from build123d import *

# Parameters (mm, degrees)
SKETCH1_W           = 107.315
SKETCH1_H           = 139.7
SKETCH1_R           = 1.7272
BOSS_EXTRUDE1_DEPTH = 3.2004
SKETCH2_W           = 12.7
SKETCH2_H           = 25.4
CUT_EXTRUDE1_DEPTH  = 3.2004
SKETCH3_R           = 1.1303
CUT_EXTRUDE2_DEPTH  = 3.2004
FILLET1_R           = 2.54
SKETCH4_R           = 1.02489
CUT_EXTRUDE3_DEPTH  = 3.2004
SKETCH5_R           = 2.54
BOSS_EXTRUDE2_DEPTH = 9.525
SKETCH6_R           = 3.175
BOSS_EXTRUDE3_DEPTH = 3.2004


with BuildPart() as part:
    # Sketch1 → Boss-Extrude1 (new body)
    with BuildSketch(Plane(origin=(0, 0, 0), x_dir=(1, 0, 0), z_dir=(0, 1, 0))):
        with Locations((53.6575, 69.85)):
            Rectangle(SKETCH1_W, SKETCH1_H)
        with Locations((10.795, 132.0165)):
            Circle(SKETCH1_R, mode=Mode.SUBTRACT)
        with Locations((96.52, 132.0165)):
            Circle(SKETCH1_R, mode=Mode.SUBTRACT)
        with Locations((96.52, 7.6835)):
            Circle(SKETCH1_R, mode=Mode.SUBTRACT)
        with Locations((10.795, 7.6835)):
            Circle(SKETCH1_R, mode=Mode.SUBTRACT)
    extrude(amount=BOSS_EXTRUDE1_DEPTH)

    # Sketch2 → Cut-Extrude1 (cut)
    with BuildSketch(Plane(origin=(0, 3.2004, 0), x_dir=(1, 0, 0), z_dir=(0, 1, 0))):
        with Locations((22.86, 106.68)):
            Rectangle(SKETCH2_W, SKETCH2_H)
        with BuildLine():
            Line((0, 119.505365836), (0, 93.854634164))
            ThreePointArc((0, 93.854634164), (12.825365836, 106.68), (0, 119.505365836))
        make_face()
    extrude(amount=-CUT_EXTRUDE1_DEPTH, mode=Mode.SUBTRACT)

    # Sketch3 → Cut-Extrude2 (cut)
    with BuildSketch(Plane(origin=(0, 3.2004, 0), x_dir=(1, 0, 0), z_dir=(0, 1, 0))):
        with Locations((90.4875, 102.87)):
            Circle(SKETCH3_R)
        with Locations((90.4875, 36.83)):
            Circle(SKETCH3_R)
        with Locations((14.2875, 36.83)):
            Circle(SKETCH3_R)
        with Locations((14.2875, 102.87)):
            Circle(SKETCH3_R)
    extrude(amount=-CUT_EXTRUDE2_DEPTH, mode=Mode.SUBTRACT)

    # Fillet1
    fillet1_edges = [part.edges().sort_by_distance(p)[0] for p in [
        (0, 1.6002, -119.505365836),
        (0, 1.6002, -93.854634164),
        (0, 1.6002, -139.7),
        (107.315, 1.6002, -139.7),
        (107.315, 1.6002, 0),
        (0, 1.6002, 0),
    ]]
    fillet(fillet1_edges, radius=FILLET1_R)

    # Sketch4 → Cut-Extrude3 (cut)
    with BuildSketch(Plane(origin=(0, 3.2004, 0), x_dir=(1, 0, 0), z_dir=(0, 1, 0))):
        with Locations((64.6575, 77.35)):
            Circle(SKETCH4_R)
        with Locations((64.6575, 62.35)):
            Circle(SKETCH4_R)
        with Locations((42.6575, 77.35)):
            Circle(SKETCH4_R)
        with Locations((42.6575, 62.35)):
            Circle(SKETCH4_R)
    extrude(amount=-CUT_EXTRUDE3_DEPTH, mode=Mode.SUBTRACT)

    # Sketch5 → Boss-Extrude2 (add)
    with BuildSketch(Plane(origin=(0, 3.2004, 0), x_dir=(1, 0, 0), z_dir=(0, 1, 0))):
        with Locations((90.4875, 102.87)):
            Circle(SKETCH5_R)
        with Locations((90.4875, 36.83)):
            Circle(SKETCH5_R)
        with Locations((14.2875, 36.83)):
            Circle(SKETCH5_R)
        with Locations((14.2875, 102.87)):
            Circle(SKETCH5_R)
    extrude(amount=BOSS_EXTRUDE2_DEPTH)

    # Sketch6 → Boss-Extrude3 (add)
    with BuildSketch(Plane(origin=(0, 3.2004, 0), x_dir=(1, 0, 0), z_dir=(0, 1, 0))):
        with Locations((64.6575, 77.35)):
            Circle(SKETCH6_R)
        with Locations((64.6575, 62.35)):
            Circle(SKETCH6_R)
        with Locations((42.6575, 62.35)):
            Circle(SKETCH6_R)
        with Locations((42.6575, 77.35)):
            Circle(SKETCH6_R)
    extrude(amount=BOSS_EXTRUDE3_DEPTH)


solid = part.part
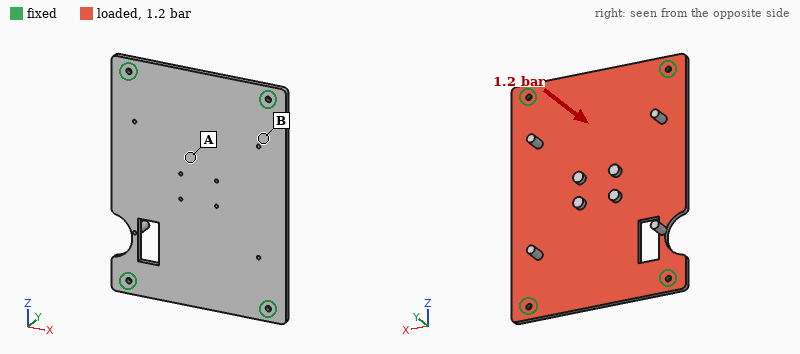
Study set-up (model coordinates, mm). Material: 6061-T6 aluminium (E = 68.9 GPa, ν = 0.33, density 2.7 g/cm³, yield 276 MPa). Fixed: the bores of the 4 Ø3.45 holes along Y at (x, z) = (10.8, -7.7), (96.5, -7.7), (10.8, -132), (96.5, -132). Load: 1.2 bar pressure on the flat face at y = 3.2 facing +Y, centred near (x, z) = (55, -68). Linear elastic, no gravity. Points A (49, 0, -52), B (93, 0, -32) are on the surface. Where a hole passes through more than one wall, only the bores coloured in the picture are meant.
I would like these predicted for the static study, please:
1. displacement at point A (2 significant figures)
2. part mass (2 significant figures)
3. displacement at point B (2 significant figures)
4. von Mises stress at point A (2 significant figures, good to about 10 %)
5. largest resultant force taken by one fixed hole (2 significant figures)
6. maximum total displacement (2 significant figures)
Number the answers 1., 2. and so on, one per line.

1. 0.58 mm
2. 130 g
3. 0.26 mm
4. 41 MPa
5. 440 N
6. 0.65 mm
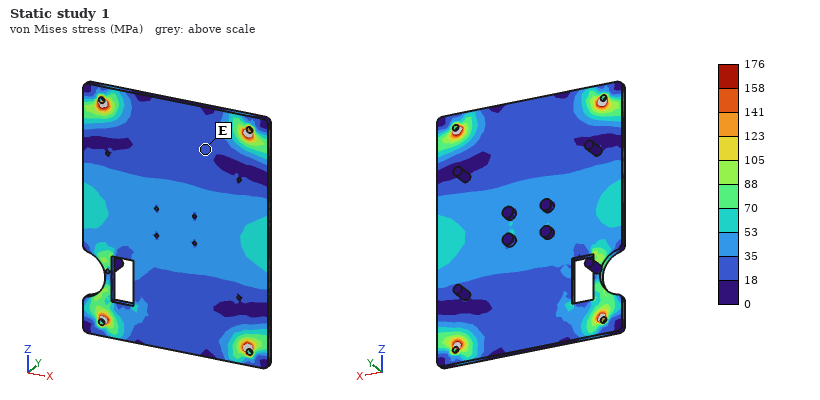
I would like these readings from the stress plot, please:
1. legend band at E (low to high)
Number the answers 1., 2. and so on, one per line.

1. 18 to 35 MPa
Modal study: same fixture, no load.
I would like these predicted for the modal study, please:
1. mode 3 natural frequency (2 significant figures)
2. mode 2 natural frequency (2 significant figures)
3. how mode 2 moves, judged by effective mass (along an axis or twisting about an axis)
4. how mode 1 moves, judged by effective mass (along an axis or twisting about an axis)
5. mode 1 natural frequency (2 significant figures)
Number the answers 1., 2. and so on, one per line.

1. 1900 Hz
2. 1200 Hz
3. twisting about Z
4. along Y
5. 820 Hz
